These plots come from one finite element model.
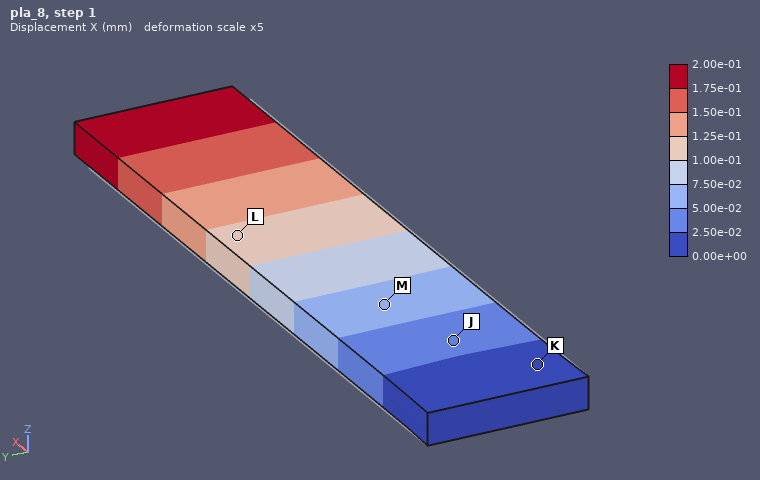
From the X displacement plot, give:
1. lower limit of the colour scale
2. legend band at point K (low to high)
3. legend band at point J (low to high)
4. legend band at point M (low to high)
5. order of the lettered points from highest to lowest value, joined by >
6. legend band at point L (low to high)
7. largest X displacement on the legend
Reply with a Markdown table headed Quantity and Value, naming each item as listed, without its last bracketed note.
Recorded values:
| Quantity | Value |
|---|---|
| lower limit of the colour scale | 0.00e+00 mm |
| legend band at point K | 0.00e+00 to 2.50e-02 mm |
| legend band at point J | 2.50e-02 to 5.00e-02 mm |
| legend band at point M | 5.00e-02 to 7.50e-02 mm |
| order of the lettered points from highest to lowest value, joined by > | L > M > J > K |
| legend band at point L | 1.00e-01 to 1.25e-01 mm |
| largest X displacement on the legend | 2.00e-01 mm |
